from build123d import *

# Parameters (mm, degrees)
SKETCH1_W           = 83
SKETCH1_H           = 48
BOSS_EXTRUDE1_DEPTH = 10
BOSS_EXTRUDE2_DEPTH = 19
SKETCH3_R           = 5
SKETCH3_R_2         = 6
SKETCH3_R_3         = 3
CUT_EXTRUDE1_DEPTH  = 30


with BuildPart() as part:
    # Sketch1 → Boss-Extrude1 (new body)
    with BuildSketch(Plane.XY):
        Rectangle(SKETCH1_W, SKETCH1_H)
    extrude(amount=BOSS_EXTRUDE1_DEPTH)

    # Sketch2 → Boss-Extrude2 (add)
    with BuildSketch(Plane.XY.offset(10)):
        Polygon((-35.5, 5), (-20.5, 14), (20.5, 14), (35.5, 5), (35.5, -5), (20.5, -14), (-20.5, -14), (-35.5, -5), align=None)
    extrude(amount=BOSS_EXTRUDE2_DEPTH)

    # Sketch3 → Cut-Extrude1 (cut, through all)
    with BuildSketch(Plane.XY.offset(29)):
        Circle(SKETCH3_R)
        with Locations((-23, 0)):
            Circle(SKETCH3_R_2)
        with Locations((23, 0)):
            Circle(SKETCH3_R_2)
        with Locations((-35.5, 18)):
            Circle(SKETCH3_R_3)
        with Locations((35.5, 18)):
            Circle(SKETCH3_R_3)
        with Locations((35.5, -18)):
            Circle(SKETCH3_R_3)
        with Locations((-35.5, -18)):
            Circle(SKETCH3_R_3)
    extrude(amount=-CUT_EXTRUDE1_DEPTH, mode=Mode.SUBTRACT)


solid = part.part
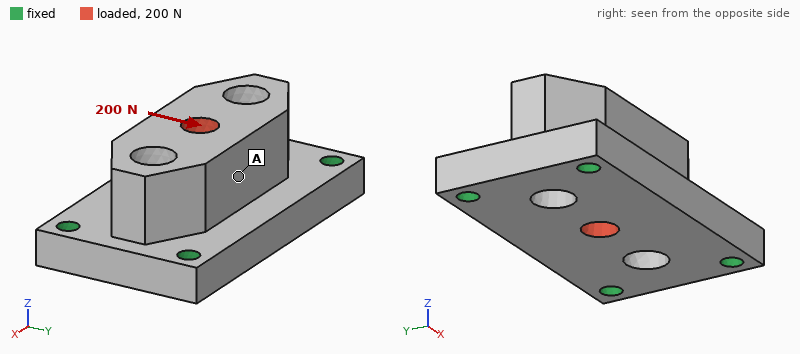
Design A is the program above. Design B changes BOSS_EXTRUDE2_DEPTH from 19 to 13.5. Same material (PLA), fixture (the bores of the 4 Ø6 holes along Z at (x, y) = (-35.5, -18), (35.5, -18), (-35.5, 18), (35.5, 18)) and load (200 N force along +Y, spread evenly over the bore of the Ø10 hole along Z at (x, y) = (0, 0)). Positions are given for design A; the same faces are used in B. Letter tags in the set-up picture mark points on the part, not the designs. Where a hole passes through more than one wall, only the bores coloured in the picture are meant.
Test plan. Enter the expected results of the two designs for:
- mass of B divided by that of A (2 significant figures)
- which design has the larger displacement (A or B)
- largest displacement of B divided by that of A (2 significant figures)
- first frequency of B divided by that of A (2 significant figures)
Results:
0.88
A
0.79
1.0
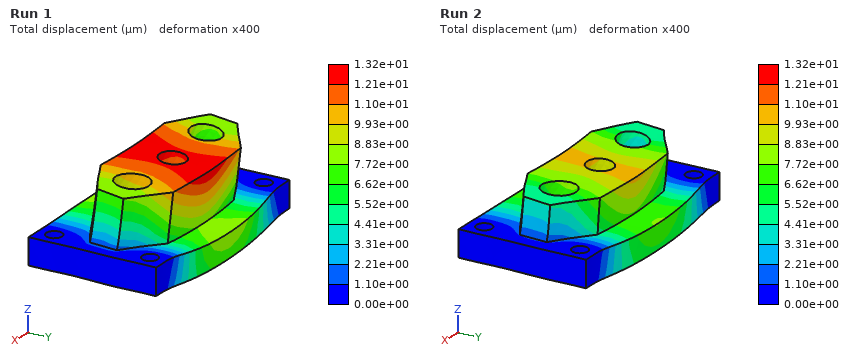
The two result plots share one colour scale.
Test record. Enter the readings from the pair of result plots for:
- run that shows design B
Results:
Run 2
